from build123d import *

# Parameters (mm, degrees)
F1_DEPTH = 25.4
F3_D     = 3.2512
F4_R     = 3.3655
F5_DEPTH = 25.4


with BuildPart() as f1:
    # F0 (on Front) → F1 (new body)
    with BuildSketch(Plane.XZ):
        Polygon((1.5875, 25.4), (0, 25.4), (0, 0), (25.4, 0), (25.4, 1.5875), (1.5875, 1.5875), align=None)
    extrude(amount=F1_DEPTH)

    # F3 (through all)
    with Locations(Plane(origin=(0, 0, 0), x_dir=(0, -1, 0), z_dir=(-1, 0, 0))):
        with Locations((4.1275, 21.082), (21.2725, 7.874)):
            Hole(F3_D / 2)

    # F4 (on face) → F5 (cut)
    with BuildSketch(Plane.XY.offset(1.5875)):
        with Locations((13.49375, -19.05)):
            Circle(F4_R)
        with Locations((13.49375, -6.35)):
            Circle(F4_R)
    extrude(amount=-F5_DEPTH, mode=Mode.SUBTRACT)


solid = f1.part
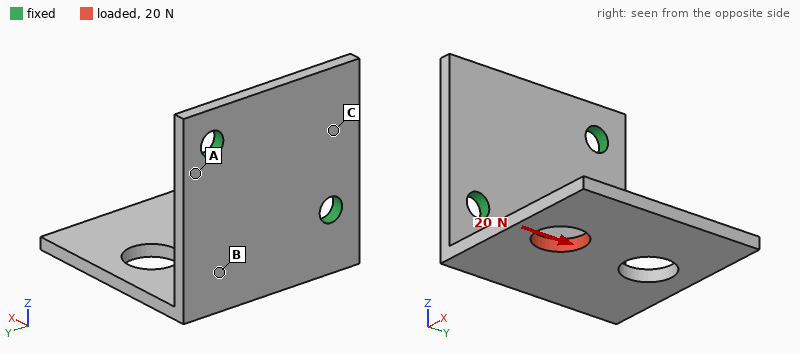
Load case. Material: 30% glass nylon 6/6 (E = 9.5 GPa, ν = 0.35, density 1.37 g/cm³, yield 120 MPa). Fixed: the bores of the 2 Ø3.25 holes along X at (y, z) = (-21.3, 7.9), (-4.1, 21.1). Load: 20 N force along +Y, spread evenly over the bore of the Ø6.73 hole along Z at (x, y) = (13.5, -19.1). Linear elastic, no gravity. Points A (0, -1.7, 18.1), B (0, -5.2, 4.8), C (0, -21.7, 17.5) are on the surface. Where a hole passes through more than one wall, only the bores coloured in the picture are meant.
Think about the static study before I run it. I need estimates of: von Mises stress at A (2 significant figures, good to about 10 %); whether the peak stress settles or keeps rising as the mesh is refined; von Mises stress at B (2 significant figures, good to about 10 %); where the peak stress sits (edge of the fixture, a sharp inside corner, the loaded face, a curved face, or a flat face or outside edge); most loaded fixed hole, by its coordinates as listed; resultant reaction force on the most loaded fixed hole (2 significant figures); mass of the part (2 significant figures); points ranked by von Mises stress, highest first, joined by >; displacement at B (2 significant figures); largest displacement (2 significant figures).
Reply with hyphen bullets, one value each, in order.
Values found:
- 14 MPa
- keeps rising
- 6.3 MPa
- edge of the fixture
- (-21.3, 7.9)
- 21 N
- 2.5 g
- A > B > C
- 0.14 mm
- 0.45 mm
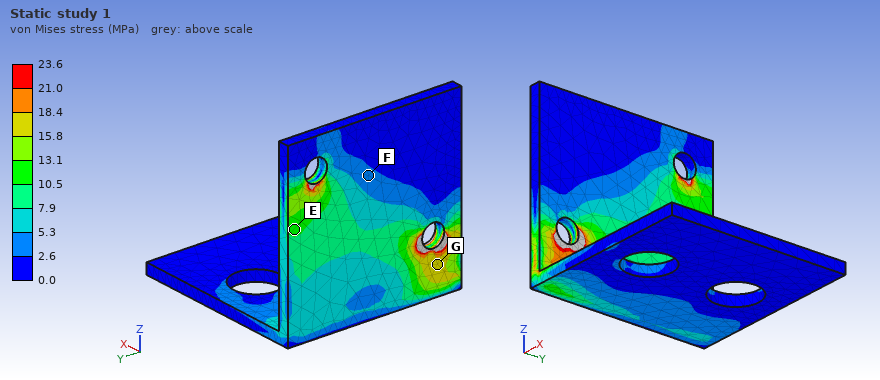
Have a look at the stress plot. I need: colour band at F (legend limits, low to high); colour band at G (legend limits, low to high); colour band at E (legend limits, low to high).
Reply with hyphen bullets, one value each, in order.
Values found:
- 2.6 to 5.3 MPa
- 15.8 to 18.4 MPa
- 10.5 to 13.1 MPa
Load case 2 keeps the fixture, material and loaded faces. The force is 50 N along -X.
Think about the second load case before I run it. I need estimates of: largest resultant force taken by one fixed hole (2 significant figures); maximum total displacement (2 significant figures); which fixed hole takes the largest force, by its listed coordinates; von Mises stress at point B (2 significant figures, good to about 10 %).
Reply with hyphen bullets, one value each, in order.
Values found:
- 51 N
- 0.49 mm
- (-21.3, 7.9)
- 5.6 MPa
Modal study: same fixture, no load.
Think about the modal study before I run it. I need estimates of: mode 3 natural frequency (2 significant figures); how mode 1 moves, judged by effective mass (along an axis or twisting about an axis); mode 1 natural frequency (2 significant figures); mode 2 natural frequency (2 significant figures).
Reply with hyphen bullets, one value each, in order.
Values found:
- 2300 Hz
- along Z
- 720 Hz
- 1200 Hz
